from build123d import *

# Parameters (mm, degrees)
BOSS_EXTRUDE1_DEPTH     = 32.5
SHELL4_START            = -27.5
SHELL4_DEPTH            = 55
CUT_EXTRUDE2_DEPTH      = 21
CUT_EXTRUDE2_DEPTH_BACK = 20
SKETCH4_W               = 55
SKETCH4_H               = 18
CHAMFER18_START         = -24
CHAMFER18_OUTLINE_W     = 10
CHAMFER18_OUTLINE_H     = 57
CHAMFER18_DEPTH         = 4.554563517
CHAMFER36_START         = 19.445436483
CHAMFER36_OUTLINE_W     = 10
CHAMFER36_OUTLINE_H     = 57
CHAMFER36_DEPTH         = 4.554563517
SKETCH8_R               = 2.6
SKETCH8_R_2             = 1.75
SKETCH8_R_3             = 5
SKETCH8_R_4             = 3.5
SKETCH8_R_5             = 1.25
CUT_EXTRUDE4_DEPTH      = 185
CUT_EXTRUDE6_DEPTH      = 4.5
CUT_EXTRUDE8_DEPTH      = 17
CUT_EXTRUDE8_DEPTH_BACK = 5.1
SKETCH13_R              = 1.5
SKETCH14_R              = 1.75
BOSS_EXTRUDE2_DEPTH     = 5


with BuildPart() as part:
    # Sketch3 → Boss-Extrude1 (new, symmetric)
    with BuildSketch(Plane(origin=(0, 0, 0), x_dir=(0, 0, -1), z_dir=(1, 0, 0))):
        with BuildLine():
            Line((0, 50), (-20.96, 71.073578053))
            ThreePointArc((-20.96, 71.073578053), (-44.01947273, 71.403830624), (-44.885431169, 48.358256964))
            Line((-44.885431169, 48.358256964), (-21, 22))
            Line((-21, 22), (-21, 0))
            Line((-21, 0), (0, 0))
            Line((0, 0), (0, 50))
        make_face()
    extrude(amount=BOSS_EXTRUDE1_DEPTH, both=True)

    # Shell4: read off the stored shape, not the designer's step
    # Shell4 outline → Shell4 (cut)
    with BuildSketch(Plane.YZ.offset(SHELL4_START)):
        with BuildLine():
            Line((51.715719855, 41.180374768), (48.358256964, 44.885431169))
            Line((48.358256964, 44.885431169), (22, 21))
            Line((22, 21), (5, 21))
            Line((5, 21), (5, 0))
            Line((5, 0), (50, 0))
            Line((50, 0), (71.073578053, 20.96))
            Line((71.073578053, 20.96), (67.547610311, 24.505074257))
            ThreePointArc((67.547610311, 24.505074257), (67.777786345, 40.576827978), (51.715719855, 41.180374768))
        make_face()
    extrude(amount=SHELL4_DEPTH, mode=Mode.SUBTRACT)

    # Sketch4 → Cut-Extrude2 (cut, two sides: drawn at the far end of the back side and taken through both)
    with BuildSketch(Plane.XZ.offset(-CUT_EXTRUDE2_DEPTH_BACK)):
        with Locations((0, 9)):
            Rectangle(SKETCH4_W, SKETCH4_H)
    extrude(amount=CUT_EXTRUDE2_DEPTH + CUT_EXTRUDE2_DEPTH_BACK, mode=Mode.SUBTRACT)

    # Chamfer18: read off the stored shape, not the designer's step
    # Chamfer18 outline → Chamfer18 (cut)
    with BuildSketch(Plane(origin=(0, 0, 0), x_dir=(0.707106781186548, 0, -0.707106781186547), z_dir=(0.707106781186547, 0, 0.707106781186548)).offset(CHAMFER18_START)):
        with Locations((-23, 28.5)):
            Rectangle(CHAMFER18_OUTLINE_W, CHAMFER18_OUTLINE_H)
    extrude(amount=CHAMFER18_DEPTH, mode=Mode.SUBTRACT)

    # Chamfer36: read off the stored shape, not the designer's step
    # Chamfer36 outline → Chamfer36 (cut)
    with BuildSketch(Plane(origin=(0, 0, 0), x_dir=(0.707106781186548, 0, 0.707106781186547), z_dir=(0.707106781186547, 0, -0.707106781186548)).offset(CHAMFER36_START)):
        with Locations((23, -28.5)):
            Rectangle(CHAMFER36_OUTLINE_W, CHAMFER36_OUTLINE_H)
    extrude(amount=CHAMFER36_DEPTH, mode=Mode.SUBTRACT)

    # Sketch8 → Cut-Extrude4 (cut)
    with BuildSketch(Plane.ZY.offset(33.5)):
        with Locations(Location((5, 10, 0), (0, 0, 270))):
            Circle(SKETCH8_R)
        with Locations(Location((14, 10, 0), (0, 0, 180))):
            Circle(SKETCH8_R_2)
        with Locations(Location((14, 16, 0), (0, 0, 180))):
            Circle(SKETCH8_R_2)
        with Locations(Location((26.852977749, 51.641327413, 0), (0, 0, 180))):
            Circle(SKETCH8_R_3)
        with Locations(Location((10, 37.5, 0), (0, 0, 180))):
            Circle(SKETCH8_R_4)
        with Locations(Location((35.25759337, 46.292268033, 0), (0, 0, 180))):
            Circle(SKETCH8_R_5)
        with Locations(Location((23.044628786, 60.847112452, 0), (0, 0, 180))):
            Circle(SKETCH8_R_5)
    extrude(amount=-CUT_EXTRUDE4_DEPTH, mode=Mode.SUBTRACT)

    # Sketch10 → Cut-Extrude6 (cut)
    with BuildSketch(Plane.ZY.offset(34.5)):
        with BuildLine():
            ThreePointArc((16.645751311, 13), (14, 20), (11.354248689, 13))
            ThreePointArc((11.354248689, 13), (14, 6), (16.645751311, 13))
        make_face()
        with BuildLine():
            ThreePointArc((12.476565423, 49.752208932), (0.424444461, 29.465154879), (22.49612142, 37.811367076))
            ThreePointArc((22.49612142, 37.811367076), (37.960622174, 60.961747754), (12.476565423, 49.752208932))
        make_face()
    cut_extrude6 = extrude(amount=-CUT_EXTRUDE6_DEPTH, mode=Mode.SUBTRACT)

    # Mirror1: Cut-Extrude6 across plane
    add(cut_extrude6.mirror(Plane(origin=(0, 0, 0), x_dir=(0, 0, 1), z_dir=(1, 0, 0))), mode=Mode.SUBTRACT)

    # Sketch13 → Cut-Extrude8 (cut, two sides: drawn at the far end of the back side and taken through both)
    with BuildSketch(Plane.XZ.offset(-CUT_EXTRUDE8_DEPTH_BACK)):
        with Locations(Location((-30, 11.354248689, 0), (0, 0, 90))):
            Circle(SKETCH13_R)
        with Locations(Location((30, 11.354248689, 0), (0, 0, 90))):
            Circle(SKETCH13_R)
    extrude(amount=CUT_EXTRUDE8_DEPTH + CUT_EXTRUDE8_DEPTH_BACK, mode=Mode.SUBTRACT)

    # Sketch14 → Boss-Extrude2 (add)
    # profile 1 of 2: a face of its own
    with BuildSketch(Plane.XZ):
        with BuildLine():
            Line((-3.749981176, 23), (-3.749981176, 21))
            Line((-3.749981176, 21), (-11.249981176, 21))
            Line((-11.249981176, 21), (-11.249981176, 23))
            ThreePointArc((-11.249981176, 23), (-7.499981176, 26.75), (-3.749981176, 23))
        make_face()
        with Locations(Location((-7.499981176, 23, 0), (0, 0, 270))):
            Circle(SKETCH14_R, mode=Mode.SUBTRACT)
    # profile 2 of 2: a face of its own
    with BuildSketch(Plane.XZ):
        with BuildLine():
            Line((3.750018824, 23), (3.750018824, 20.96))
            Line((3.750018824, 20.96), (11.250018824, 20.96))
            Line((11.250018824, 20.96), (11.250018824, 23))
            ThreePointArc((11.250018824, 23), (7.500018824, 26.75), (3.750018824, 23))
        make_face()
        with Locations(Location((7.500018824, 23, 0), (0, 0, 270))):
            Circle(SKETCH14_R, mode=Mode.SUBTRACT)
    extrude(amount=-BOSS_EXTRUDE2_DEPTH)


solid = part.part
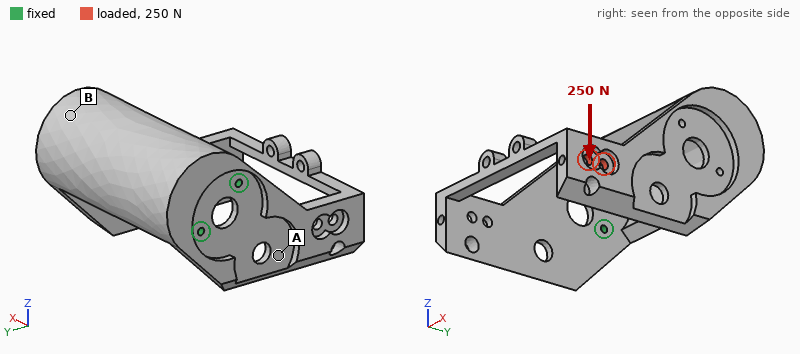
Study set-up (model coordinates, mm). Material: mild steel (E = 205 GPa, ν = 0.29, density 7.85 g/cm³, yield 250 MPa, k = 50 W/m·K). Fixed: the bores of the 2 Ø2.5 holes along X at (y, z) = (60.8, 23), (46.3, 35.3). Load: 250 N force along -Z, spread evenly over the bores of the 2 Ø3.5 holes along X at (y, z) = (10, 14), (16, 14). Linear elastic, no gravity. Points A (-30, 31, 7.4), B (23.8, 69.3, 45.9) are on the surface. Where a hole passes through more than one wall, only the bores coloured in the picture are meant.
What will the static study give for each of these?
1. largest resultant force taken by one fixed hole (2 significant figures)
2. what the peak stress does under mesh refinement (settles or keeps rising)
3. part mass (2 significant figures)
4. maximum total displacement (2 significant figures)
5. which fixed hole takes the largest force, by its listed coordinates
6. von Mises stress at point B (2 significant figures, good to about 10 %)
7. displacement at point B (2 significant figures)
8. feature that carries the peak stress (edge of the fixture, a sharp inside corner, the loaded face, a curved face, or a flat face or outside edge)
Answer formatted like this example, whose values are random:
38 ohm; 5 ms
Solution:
710 N; keeps rising; 220 g; 0.67 mm; (46.3, 35.3); 36 MPa; 0.35 mm; edge of the fixture
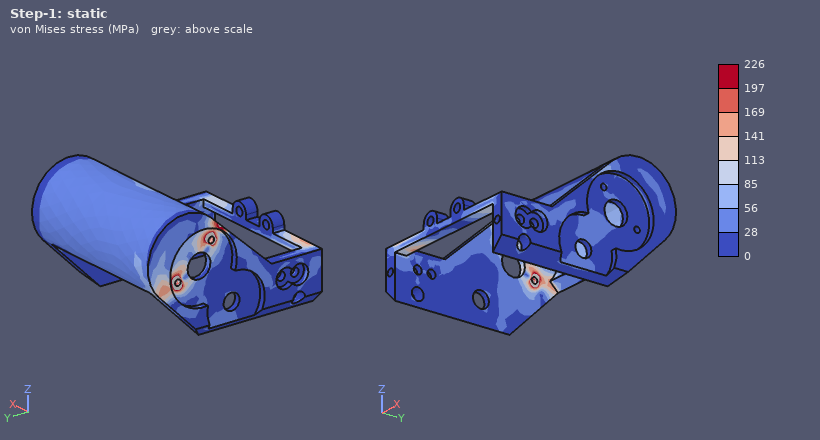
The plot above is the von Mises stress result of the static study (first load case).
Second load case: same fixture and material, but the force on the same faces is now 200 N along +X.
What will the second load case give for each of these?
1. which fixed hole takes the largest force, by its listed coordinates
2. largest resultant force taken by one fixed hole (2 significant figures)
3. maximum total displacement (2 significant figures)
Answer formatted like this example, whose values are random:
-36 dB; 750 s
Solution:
(46.3, 35.3); 270 N; 0.42 mm
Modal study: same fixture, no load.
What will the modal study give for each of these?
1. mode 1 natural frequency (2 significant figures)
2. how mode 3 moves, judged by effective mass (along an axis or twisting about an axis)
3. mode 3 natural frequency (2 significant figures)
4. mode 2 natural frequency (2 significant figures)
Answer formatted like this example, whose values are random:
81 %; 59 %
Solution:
340 Hz; along X; 980 Hz; 630 Hz
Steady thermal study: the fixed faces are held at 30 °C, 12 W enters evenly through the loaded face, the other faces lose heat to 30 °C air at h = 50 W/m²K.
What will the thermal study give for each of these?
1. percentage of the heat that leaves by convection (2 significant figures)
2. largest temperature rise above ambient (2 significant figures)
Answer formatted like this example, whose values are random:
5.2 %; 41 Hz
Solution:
94 %; 80 K
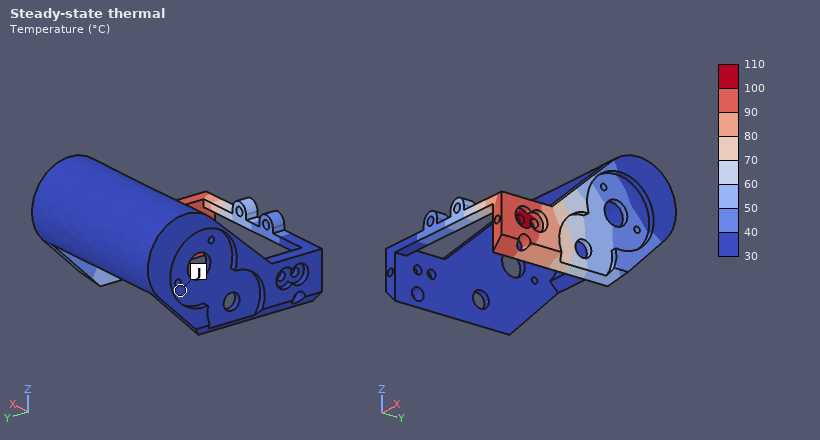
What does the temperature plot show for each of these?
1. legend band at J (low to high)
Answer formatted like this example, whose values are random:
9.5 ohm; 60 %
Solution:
30 to 40 °C
